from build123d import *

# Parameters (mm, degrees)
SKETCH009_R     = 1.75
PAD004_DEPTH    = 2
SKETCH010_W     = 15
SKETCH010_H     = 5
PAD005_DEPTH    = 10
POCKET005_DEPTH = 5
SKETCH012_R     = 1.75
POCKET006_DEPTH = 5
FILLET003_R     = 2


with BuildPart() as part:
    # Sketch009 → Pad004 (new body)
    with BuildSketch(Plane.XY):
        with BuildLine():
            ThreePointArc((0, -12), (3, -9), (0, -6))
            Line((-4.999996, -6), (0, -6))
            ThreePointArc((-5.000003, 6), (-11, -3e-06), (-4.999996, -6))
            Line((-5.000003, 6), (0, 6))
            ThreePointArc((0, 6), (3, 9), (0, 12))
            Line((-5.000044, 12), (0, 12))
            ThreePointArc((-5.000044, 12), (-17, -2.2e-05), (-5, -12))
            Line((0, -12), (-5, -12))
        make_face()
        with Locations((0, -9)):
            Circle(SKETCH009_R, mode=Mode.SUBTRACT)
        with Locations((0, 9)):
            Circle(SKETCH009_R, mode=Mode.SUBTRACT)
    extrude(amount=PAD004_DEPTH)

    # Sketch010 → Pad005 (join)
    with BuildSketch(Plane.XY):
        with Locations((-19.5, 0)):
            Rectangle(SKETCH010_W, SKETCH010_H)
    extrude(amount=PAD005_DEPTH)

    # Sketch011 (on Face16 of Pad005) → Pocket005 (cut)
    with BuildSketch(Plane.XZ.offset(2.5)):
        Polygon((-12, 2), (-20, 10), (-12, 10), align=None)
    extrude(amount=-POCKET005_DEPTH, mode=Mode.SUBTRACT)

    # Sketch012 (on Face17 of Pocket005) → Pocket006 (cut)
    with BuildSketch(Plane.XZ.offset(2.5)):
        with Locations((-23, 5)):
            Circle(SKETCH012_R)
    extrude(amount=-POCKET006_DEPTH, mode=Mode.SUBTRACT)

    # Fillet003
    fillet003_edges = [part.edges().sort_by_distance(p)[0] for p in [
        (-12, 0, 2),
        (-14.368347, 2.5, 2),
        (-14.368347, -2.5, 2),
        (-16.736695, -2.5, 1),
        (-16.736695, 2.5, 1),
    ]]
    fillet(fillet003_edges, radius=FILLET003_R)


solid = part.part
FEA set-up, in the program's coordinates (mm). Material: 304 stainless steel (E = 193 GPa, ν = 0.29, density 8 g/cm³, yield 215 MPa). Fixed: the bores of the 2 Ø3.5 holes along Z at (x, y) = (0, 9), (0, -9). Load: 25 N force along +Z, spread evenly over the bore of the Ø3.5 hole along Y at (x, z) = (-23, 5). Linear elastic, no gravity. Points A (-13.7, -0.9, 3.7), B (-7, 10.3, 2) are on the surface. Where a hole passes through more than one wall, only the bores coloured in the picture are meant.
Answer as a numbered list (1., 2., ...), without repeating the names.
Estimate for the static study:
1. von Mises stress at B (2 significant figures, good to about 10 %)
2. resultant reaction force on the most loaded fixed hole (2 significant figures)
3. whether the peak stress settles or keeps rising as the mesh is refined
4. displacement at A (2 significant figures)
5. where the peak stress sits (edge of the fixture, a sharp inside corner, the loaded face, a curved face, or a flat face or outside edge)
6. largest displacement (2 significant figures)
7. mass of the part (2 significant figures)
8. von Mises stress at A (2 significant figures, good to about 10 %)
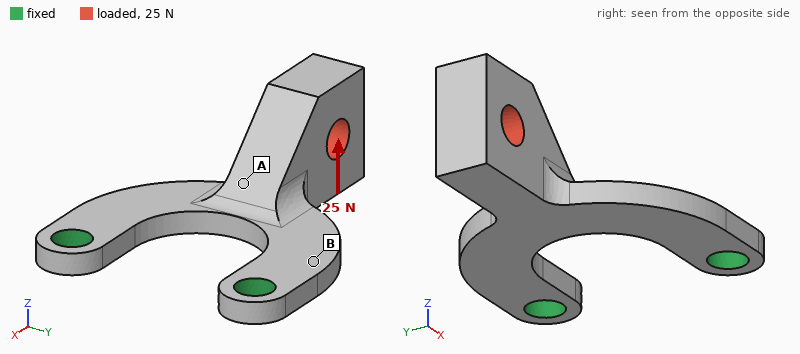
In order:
1. 47 MPa
2. 13 N
3. keeps rising
4. 25 µm
5. edge of the fixture
6. 76 µm
7. 7.8 g
8. 13 MPa
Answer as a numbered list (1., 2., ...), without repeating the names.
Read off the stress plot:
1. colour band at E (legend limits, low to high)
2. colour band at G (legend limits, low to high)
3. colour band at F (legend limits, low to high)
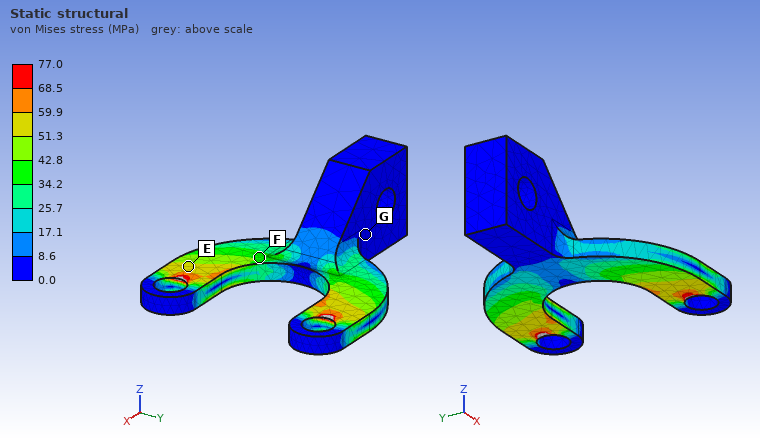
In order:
1. 51.3 to 59.9 MPa
2. 0.0 to 8.6 MPa
3. 34.2 to 42.8 MPa
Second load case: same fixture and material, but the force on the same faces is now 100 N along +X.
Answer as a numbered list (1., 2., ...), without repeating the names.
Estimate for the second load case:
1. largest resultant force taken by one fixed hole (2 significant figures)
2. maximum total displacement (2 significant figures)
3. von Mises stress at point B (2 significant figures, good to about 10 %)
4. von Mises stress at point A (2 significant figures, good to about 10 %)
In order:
1. 55 N
2. 78 µm
3. 46 MPa
4. 19 MPa
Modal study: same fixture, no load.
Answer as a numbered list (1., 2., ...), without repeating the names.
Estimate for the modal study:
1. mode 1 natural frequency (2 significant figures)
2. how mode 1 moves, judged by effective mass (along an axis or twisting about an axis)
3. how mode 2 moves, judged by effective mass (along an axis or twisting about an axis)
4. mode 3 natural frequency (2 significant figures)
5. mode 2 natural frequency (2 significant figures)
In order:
1. 1700 Hz
2. along Z
3. along Y
4. 11 kHz
5. 7700 Hz
